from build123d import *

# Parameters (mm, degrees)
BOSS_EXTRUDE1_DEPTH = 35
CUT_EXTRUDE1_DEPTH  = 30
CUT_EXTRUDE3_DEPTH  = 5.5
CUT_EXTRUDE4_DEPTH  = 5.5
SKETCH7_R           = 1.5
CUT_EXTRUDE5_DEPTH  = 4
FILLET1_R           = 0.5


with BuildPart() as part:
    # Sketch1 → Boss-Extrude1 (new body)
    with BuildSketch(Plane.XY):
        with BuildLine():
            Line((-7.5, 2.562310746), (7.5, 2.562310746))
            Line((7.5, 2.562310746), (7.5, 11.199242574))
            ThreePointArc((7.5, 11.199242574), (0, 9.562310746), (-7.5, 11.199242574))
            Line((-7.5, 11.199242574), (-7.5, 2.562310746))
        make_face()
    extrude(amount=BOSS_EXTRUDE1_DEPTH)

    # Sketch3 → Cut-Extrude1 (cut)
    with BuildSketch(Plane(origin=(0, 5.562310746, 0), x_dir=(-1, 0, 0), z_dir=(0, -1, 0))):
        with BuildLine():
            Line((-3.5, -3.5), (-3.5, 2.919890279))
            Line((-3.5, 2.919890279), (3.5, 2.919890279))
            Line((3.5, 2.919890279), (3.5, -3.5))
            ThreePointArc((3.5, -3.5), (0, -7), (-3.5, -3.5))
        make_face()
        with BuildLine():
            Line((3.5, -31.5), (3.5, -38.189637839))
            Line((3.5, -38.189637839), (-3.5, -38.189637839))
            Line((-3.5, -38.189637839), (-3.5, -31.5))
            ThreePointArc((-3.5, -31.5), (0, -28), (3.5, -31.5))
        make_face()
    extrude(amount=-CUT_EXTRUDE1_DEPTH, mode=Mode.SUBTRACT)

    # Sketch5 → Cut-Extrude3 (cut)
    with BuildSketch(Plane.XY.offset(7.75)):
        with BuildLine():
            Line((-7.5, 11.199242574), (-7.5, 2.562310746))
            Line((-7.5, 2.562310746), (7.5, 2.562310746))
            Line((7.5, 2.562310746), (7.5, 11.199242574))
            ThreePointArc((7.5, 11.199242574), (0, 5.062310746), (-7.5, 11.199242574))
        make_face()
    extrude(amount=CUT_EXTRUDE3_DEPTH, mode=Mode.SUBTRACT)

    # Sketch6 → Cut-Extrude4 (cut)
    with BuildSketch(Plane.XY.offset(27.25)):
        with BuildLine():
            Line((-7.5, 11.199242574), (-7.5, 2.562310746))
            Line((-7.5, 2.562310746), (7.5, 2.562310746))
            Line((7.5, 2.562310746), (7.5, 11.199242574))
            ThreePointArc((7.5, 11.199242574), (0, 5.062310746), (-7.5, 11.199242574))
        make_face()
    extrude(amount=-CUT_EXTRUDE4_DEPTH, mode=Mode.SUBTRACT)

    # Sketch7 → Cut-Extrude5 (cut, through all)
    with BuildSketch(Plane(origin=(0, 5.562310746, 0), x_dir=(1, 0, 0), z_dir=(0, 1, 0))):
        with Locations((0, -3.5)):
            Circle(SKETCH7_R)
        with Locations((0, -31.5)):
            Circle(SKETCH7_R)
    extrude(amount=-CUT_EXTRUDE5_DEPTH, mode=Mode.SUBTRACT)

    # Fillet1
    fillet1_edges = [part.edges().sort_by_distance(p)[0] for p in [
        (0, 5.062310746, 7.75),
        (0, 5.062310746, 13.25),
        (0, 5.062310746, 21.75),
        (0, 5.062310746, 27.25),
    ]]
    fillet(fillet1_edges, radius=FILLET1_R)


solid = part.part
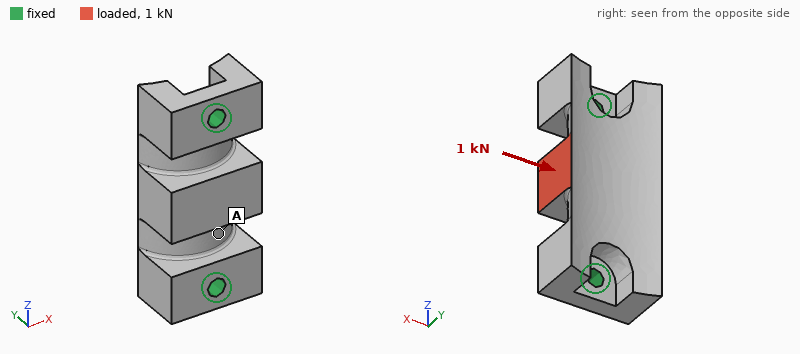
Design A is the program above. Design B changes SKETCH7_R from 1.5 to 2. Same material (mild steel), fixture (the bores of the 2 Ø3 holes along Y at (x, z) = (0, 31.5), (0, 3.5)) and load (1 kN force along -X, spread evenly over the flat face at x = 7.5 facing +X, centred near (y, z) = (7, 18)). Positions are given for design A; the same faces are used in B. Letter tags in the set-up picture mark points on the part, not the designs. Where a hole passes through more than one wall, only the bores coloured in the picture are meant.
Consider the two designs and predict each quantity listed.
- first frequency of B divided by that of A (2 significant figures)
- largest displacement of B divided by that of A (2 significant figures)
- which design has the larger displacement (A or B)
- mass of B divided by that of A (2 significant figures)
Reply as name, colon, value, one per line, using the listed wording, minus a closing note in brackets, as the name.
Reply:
first frequency of B divided by that of A: 1.2
largest displacement of B divided by that of A: 0.75
which design has the larger displacement: A
mass of B divided by that of A: 0.99
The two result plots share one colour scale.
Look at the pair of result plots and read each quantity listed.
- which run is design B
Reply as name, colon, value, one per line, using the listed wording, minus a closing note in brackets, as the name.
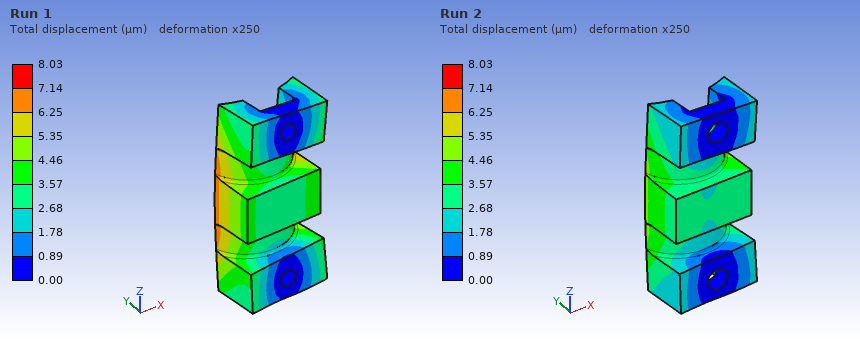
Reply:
which run is design B: Run 2
